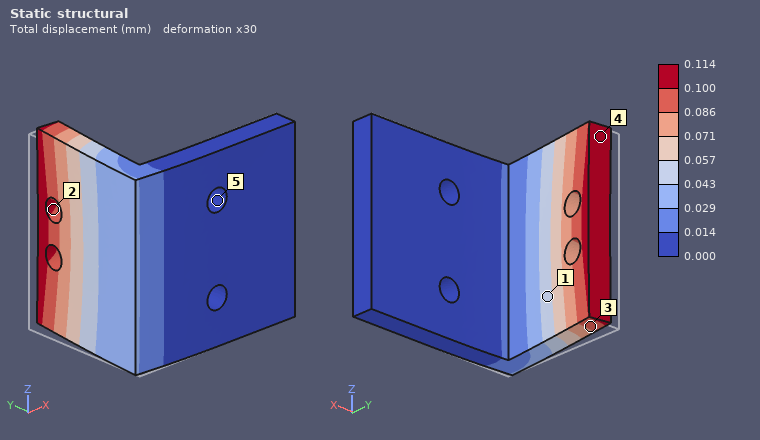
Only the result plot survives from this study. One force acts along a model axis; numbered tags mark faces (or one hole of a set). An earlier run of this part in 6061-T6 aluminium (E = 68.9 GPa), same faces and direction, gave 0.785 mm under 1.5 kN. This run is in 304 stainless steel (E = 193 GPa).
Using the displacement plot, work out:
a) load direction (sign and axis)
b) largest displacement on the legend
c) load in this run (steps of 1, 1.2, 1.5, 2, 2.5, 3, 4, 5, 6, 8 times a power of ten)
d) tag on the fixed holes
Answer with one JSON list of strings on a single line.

["+X", "0.114 mm", "600 N", "5"]
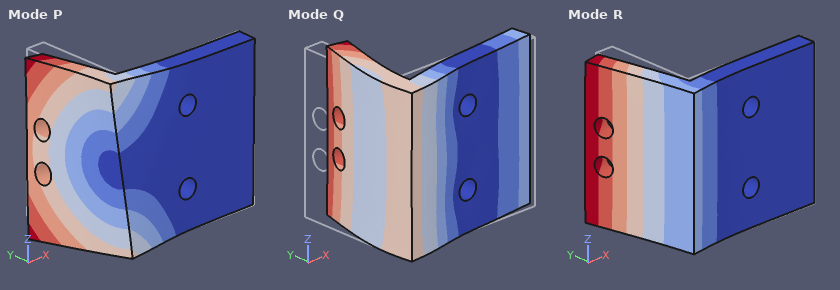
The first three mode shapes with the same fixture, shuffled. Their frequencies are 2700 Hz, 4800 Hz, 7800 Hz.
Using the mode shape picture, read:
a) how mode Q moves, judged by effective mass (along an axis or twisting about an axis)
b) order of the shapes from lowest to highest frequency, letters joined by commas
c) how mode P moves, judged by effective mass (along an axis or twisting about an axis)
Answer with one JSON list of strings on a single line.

["along Y", "R, P, Q", "along Z"]
